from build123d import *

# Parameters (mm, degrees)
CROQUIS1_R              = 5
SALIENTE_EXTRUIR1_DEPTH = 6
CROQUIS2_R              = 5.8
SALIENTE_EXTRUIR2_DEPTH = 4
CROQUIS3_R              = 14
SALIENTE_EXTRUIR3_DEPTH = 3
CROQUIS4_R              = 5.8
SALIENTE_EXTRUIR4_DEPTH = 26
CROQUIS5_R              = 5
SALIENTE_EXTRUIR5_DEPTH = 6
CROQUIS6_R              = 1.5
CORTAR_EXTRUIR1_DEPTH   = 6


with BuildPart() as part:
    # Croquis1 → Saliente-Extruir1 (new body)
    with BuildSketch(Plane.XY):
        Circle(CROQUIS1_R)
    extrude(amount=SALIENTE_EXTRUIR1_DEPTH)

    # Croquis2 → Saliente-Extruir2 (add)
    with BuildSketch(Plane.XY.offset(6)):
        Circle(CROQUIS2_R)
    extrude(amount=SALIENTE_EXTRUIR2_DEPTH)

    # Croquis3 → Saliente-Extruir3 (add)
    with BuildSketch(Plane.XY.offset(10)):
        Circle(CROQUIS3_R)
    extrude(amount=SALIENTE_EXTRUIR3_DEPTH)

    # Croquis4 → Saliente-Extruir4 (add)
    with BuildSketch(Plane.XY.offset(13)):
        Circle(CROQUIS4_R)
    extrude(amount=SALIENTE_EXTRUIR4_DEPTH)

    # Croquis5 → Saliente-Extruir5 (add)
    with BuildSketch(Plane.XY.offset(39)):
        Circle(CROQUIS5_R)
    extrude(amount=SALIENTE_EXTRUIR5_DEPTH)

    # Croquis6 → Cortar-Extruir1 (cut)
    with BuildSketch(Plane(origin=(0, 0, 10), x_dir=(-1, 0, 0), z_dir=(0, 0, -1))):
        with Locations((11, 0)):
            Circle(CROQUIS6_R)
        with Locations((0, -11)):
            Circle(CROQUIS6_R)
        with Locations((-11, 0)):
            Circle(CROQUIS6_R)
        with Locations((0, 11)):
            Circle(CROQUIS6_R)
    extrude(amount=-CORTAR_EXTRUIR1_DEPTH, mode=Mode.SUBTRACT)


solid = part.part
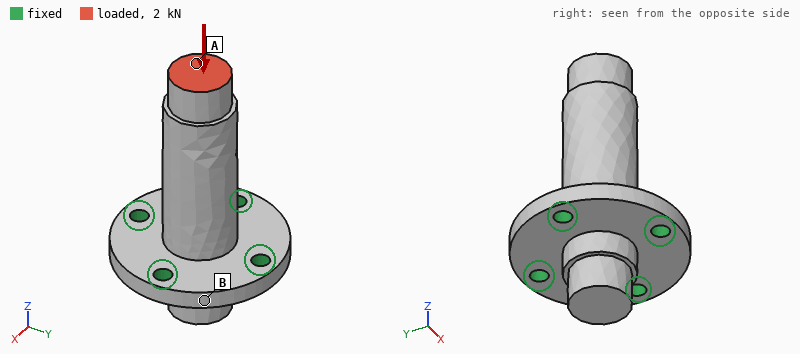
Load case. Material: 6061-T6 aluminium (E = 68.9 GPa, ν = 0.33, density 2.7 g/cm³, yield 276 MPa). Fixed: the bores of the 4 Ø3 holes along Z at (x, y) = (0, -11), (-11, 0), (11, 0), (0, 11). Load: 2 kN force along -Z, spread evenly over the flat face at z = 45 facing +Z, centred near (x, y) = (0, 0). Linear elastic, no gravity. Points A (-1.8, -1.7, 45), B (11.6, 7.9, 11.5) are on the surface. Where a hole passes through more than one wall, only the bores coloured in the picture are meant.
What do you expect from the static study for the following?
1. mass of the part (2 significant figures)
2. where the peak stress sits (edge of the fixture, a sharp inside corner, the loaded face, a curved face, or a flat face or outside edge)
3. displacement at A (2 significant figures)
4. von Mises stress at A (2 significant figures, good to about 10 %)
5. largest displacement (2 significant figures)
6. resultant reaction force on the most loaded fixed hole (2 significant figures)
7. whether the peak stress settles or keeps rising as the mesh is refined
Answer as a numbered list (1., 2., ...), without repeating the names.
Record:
1. 16 g
2. edge of the fixture
3. 18 µm
4. 26 MPa
5. 18 µm
6. 500 N
7. keeps rising
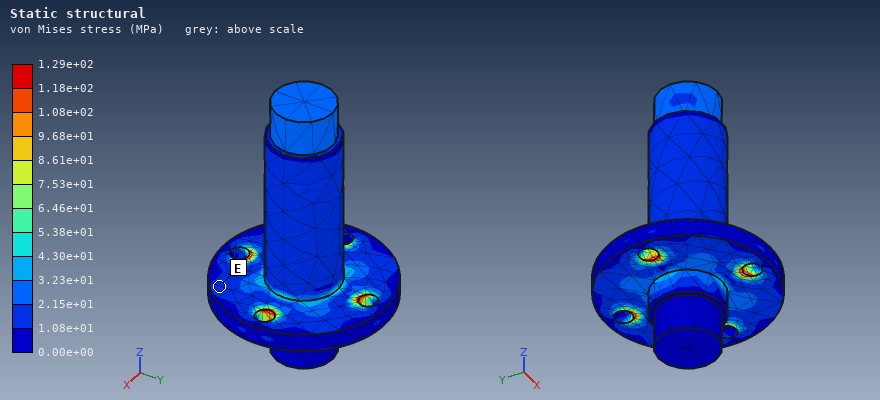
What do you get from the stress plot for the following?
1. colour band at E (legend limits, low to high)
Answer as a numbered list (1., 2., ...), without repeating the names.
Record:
1. 1.08e+01 to 2.15e+01 MPa
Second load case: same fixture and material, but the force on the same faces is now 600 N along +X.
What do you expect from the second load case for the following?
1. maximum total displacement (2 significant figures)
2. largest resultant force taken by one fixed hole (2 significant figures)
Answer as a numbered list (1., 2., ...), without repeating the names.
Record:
1. 0.21 mm
2. 1.1 kN
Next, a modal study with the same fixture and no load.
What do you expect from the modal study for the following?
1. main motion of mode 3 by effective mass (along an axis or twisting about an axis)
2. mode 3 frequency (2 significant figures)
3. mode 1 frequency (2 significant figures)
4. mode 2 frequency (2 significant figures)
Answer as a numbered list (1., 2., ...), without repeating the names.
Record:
1. along Z
2. 20 kHz
3. 5600 Hz
4. 5600 Hz
